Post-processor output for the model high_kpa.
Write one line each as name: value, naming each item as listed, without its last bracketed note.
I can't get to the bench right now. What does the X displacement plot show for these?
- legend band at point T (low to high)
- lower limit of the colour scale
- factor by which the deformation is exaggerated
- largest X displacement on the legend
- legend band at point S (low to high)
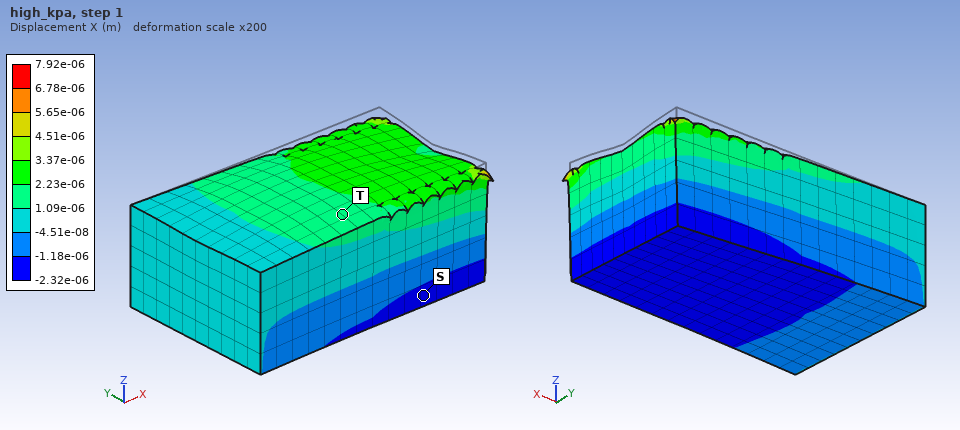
legend band at point T: 1.09e-06 to 2.23e-06 m
lower limit of the colour scale: -2.32e-06 m
factor by which the deformation is exaggerated: 200
largest X displacement on the legend: 7.92e-06 m
legend band at point S: -2.32e-06 to -1.18e-06 m
